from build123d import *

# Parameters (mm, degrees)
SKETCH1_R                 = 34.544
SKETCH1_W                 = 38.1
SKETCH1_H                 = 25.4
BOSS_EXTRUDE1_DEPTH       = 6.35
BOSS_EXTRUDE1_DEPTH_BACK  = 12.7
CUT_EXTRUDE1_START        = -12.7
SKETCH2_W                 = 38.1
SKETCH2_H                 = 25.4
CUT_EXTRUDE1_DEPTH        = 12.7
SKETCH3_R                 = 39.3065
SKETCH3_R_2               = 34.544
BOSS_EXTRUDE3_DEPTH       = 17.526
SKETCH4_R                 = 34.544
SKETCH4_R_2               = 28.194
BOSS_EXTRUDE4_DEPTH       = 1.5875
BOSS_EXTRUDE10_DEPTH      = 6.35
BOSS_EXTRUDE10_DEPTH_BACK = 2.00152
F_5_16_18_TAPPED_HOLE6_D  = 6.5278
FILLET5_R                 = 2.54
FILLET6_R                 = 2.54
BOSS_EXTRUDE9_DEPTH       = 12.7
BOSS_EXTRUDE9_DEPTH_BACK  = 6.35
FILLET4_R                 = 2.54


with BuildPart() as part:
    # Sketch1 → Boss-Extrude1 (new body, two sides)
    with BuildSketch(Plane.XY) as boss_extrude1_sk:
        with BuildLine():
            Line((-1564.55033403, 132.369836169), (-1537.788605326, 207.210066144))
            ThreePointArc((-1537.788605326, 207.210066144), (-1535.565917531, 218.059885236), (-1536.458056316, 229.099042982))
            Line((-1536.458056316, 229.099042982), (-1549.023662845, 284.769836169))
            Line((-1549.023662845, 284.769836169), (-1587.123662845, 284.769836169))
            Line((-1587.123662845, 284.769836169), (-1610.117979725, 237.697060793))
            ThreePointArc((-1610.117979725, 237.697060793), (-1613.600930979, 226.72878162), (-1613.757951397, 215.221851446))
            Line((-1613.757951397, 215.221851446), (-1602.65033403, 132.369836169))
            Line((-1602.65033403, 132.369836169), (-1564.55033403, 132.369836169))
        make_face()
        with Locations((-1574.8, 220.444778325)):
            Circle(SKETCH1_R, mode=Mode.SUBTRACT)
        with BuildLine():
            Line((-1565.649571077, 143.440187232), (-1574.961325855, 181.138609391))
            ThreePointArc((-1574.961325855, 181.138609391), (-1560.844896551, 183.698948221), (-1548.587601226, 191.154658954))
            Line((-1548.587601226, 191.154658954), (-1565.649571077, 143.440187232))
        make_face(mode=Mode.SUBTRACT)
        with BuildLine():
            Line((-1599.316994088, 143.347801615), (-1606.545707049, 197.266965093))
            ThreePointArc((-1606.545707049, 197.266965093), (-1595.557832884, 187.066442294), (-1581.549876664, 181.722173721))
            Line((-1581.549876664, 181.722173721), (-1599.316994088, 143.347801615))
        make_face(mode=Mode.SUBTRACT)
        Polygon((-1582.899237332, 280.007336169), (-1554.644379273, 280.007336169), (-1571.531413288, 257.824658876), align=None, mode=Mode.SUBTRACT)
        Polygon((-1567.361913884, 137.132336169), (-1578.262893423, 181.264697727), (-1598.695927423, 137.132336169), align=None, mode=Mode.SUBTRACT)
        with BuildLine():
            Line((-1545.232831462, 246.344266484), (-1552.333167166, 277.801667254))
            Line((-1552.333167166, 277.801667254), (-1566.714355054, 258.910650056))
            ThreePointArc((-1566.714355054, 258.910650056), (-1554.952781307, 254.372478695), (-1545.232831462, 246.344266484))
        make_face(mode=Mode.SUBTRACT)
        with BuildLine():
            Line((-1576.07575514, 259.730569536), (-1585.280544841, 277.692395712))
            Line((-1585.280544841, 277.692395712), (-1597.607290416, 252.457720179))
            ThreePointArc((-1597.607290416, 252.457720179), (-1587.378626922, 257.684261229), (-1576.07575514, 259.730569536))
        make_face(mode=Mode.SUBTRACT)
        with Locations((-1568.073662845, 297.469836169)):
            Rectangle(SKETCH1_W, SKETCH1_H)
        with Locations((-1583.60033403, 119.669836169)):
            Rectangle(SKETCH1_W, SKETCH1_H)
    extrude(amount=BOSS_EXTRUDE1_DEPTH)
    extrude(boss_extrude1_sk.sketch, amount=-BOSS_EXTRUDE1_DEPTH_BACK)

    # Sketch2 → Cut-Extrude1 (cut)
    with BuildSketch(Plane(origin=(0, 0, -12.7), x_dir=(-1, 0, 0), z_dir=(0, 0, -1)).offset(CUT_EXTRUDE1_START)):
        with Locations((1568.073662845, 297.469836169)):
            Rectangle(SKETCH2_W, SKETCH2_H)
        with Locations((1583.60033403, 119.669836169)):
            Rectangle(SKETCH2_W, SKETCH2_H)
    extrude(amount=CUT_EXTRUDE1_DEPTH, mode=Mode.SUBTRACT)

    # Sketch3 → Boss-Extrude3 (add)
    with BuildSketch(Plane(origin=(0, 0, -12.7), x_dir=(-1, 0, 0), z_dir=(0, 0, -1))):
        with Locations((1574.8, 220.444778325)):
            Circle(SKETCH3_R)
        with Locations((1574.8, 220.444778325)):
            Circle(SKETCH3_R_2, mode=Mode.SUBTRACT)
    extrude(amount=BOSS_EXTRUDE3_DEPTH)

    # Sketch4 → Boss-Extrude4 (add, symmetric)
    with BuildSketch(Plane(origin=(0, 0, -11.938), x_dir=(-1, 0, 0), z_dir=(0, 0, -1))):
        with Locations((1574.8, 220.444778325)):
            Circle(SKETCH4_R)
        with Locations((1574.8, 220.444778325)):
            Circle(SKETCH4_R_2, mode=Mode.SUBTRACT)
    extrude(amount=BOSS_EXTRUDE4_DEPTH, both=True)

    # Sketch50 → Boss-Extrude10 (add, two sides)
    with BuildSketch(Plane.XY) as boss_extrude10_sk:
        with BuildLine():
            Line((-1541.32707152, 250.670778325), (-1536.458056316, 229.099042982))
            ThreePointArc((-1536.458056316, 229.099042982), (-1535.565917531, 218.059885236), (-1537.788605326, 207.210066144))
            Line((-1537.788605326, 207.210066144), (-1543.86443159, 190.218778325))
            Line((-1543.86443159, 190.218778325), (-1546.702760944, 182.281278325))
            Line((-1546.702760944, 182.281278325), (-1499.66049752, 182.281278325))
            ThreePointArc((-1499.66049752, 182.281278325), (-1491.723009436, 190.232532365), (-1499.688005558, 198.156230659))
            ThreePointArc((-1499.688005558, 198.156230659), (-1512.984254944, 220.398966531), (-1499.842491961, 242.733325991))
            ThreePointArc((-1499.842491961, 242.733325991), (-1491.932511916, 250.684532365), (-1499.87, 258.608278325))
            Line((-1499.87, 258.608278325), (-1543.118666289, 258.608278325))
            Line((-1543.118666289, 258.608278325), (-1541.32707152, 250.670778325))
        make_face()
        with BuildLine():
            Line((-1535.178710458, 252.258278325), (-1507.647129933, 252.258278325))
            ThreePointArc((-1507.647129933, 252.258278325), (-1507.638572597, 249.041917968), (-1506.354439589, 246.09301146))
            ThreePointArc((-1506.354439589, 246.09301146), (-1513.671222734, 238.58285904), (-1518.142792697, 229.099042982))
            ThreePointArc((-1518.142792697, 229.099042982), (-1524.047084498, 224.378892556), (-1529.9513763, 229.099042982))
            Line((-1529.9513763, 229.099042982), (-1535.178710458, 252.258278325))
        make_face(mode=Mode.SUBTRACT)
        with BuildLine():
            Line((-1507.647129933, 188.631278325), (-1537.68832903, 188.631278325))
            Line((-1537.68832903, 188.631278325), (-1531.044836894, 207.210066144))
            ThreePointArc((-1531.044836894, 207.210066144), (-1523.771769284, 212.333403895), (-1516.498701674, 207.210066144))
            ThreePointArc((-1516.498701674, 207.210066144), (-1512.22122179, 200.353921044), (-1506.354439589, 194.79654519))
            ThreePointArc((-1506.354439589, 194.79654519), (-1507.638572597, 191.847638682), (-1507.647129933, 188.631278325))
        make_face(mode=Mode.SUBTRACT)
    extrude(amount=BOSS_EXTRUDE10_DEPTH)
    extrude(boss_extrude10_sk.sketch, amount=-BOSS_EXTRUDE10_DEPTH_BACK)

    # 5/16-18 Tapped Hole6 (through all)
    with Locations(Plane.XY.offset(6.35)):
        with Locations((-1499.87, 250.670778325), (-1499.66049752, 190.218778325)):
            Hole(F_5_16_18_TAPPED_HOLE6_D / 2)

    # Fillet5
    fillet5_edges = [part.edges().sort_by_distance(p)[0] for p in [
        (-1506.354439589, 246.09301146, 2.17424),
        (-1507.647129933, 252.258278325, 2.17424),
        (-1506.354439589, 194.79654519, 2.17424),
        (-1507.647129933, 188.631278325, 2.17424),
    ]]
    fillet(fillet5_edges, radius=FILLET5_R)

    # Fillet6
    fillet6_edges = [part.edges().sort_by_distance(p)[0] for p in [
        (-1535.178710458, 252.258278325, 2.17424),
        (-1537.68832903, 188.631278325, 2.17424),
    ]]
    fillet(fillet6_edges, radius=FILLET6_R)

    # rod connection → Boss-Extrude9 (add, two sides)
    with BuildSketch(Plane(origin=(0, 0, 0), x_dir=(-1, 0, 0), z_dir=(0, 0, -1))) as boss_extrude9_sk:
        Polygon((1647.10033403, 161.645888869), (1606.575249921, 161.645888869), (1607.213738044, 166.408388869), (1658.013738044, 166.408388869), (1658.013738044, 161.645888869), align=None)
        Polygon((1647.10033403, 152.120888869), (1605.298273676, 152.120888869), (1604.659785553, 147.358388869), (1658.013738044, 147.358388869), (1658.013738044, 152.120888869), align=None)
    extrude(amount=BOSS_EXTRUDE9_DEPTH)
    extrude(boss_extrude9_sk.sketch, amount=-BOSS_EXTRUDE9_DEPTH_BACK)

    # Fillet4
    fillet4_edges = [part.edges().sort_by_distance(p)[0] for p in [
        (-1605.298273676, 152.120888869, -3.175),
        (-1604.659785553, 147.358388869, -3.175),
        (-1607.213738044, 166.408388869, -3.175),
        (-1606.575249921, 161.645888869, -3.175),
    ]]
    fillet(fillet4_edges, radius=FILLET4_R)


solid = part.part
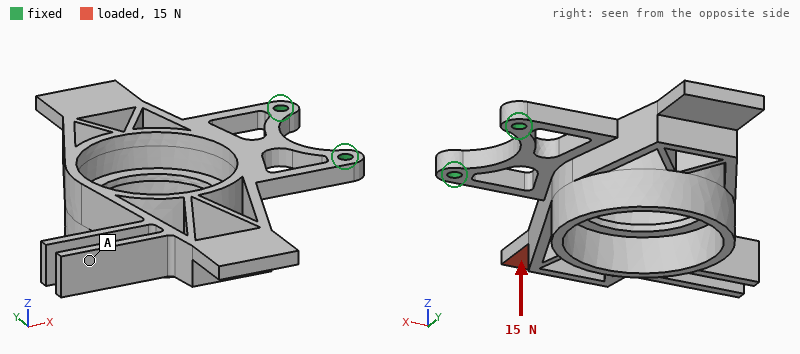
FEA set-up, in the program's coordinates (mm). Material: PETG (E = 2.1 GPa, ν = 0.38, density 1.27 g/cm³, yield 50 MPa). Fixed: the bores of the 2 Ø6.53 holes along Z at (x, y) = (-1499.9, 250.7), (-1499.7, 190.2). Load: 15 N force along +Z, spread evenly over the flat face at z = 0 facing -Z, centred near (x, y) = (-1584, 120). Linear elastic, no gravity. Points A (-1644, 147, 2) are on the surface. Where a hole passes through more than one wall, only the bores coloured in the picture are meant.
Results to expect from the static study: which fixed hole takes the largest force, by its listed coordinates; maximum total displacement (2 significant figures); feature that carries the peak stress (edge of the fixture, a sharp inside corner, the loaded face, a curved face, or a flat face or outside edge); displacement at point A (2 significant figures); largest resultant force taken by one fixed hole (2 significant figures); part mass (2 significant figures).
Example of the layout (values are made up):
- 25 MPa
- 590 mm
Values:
- (-1499.7, 190.2)
- 3.2 mm
- a curved face
- 2.9 mm
- 31 N
- 150 g
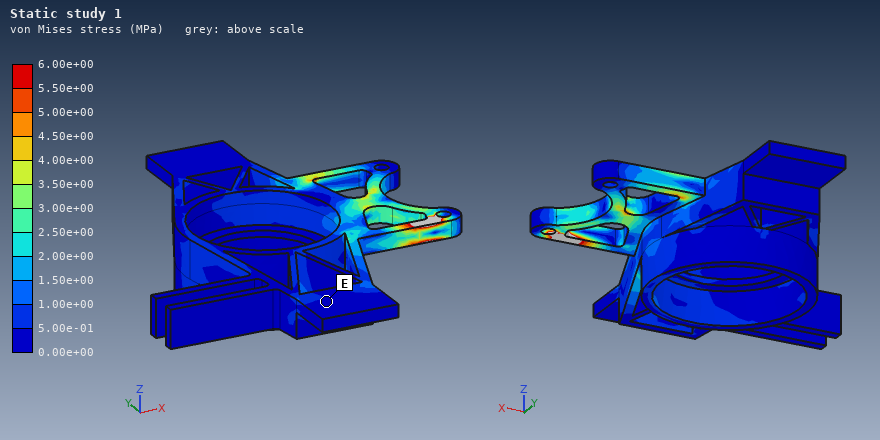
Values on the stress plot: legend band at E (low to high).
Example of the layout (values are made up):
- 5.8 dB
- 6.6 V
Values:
- 0.00e+00 to 5.00e-01 MPa
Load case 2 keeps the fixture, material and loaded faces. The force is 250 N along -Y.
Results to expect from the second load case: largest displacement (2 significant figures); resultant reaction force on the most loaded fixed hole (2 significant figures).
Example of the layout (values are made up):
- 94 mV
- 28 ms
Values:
- 2.8 mm
- 340 N
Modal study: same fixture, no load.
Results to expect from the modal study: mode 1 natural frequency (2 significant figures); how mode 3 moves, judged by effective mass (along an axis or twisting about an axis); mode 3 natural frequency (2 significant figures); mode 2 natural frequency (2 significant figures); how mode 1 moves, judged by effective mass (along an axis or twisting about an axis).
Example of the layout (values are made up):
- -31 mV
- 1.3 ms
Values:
- 47 Hz
- along Y
- 170 Hz
- 120 Hz
- along Z
